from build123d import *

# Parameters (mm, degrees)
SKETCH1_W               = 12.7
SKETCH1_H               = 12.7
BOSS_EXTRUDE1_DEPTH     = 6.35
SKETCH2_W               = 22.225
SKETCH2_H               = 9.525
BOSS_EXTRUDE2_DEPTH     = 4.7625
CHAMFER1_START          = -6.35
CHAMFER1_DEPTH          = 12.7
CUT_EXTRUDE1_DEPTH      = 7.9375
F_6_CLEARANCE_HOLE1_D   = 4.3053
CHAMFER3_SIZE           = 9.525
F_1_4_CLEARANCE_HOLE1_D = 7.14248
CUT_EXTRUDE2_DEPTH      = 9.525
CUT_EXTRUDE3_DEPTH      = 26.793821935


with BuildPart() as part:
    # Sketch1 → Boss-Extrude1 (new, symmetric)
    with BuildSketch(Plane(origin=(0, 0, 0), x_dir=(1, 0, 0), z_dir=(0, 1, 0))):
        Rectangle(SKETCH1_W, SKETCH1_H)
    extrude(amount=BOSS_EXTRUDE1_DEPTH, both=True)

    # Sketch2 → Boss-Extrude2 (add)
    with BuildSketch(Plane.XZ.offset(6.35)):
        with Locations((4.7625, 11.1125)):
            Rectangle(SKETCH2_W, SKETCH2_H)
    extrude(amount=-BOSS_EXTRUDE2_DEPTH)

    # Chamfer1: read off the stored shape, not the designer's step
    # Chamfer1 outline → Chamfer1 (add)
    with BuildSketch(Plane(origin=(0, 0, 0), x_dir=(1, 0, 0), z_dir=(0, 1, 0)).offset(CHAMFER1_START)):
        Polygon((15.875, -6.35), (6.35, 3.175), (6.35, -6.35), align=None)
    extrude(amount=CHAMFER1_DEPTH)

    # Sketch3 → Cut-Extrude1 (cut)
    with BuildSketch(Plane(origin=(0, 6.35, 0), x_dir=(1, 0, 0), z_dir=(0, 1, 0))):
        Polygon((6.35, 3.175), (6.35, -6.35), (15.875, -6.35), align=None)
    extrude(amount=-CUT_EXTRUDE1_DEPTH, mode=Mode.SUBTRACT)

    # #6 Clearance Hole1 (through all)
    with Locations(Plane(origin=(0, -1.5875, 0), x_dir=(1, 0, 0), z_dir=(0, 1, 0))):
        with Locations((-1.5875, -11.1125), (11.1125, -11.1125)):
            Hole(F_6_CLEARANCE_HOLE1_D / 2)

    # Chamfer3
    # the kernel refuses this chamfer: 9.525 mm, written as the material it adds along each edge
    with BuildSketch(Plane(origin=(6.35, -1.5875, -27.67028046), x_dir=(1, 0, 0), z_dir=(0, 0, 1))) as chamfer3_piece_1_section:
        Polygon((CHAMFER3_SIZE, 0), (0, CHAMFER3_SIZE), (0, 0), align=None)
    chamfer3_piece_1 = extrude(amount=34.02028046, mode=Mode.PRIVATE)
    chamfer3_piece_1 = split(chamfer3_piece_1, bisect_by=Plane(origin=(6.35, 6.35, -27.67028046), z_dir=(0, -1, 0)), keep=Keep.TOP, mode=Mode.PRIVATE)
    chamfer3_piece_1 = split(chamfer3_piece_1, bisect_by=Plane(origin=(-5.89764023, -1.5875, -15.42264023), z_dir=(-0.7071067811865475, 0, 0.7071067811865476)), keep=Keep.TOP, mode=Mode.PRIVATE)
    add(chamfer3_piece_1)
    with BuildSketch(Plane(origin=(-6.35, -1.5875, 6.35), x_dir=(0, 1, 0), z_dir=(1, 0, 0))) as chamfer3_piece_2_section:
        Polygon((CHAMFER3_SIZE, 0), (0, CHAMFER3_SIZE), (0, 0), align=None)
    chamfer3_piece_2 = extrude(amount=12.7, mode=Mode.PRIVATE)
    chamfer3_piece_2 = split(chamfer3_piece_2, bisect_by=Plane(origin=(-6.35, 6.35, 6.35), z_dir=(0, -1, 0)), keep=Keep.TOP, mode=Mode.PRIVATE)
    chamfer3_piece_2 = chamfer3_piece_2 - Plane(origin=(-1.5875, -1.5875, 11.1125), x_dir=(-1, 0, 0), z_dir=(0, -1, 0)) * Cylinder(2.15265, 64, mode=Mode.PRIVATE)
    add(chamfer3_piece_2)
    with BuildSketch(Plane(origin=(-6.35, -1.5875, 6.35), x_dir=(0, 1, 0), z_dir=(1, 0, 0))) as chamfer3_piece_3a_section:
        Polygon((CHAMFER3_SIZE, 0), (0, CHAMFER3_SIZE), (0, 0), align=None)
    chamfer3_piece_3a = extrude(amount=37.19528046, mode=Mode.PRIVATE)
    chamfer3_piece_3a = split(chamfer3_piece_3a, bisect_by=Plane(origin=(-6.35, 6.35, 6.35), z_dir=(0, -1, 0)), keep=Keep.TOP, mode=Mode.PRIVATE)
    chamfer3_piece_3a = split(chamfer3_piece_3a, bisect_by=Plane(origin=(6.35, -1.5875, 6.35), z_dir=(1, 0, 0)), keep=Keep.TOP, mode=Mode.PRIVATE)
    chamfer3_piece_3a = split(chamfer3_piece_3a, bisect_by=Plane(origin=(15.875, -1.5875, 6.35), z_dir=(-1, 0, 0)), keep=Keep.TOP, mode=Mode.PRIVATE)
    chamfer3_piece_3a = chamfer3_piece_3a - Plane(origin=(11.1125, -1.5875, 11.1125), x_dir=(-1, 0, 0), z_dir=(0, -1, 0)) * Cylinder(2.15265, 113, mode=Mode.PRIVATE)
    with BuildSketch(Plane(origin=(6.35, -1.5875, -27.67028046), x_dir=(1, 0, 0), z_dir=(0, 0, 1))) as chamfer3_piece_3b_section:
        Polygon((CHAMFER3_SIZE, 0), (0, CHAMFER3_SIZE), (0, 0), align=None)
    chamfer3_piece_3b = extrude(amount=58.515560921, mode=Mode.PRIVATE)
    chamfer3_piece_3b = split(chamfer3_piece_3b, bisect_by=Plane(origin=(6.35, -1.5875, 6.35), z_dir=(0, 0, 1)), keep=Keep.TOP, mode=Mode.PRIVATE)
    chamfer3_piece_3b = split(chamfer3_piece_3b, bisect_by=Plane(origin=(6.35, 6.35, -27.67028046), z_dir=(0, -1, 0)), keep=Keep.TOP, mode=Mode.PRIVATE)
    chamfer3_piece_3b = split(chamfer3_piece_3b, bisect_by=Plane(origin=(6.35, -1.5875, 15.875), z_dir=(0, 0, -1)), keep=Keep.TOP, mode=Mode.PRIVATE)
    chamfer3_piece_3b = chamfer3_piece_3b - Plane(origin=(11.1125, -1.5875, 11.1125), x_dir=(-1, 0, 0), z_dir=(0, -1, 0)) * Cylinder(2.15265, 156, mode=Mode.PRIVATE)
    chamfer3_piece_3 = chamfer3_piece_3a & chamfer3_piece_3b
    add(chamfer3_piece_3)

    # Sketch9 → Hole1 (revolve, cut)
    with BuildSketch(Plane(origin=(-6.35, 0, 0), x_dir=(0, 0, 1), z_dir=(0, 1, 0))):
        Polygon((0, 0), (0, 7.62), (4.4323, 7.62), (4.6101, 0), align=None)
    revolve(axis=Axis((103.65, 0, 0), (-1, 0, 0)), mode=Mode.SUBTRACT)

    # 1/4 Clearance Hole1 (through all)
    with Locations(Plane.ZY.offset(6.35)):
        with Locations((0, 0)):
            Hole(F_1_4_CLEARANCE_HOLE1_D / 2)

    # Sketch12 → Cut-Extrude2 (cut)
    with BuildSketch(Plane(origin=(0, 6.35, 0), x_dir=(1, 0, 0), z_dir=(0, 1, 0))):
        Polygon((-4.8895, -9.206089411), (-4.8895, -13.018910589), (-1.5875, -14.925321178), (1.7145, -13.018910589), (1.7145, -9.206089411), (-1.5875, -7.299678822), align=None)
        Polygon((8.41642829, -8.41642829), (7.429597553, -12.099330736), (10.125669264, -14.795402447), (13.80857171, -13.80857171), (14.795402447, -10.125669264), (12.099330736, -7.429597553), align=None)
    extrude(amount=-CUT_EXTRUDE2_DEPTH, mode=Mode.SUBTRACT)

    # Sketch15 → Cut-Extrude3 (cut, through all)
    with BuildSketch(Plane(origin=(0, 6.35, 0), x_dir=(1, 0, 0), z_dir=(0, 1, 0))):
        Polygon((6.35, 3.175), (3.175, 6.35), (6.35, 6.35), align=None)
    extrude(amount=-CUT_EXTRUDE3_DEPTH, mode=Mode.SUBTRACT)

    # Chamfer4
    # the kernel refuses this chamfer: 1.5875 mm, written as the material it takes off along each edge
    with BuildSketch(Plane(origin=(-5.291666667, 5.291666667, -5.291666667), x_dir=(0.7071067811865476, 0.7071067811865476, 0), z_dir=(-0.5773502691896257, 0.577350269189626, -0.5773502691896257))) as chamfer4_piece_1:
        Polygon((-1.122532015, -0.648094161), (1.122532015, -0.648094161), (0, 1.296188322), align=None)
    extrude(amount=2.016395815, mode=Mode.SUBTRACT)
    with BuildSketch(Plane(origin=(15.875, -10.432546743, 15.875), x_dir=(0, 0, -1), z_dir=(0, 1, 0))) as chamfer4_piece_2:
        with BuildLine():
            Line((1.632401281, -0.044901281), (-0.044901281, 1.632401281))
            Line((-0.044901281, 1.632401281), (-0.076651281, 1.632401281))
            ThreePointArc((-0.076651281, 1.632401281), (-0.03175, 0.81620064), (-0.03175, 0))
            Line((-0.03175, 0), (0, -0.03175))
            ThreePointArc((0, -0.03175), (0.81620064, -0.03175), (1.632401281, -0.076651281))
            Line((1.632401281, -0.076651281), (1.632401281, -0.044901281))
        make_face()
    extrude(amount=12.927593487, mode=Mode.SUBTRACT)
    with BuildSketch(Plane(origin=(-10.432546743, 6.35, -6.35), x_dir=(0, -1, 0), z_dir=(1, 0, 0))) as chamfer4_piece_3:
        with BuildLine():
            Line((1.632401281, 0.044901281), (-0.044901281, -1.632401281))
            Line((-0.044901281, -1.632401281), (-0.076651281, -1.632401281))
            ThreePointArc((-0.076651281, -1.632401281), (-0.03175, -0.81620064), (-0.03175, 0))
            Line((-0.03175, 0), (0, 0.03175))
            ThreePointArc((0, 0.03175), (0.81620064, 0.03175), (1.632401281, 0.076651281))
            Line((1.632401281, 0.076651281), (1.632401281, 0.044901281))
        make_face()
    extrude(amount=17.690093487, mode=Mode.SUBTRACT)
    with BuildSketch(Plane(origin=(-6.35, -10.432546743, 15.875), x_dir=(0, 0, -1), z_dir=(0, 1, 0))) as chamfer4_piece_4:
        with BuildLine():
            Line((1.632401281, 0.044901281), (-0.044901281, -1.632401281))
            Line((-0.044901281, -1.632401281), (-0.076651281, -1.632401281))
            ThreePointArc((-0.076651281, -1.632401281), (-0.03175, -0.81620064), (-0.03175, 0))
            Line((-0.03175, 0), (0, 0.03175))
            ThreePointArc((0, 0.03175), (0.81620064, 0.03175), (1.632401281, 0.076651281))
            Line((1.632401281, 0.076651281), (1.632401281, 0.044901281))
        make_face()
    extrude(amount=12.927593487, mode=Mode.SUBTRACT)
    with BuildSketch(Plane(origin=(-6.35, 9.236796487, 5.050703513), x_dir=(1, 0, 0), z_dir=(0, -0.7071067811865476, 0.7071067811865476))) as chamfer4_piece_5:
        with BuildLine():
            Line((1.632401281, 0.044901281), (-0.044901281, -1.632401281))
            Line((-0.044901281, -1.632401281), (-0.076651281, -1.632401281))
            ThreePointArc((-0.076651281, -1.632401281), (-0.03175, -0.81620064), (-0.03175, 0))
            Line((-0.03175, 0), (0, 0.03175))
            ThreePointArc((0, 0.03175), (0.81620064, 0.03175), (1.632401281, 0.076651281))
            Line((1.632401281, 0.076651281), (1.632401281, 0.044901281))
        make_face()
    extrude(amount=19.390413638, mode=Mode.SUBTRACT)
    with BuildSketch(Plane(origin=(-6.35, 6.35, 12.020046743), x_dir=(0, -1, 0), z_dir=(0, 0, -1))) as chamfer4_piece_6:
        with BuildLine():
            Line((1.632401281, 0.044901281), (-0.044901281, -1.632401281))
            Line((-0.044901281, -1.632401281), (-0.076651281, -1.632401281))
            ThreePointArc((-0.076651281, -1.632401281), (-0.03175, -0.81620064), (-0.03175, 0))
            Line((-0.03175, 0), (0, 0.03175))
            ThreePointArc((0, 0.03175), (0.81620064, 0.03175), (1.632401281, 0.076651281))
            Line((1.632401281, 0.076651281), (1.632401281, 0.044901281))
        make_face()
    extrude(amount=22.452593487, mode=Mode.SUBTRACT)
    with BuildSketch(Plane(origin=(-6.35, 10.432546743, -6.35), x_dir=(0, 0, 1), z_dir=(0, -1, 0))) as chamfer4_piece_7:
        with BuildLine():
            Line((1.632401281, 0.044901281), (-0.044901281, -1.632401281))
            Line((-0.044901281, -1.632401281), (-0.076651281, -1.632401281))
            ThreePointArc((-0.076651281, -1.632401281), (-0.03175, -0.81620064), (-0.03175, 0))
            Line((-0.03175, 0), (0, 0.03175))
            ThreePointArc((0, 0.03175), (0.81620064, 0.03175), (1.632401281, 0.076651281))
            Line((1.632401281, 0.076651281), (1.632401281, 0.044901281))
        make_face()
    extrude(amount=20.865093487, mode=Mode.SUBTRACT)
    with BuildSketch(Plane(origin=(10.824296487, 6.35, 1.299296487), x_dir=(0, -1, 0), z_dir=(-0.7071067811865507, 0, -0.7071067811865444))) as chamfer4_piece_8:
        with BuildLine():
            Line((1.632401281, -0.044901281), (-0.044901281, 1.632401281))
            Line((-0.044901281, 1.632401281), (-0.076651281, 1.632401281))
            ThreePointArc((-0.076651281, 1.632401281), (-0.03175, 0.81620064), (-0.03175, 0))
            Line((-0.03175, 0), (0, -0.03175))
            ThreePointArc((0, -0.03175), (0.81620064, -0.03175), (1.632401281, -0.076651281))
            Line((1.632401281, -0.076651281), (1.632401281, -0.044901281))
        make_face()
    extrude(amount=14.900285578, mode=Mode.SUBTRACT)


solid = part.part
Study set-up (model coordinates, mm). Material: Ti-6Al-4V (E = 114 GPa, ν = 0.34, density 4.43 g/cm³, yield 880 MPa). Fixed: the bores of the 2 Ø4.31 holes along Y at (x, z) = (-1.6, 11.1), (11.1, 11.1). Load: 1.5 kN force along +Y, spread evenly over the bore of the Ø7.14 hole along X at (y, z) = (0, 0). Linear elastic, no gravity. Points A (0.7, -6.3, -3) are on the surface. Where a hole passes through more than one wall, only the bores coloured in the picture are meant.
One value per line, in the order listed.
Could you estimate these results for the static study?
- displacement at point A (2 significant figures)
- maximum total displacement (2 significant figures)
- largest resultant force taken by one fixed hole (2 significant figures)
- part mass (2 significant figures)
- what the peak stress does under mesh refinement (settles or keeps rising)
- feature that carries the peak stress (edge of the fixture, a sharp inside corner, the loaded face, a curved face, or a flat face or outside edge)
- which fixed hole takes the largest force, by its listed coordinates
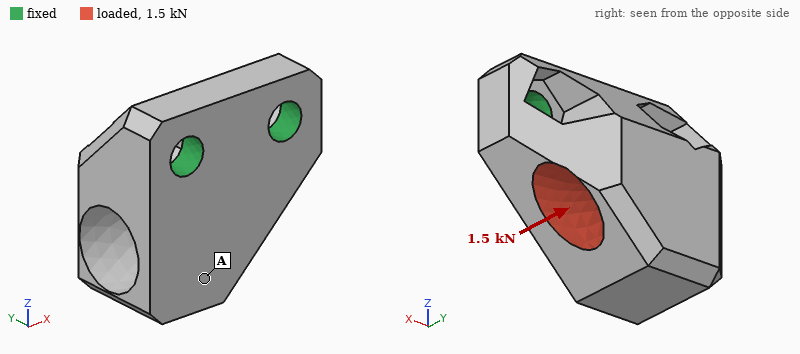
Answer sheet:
35 µm
49 µm
860 N
13 g
keeps rising
edge of the fixture
(11.1, 11.1)
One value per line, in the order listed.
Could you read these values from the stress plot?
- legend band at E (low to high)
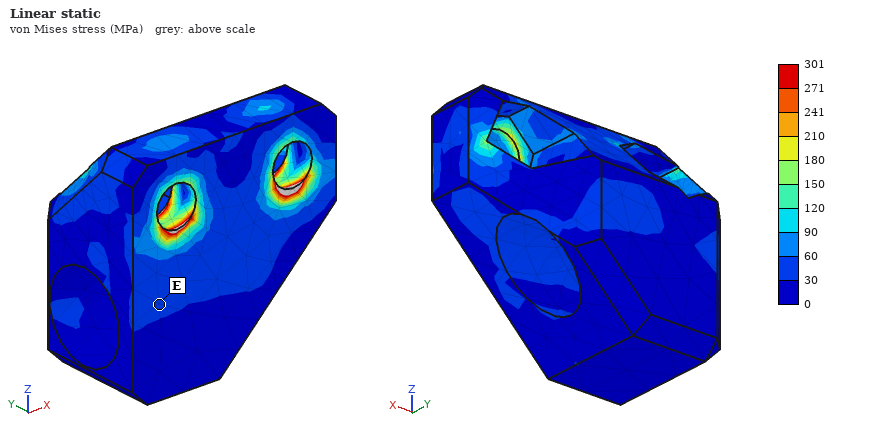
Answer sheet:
30 to 60 MPa
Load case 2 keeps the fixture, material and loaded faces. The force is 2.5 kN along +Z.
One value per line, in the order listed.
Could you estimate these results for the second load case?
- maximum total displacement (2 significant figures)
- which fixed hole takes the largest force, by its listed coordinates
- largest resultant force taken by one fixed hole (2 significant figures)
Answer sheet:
35 µm
(11.1, 11.1)
1.5 kN
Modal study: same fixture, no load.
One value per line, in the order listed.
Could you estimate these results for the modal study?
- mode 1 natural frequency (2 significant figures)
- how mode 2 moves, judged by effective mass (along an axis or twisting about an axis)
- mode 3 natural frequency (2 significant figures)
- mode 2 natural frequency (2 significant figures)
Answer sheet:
12 kHz
along X
35 kHz
26 kHz
